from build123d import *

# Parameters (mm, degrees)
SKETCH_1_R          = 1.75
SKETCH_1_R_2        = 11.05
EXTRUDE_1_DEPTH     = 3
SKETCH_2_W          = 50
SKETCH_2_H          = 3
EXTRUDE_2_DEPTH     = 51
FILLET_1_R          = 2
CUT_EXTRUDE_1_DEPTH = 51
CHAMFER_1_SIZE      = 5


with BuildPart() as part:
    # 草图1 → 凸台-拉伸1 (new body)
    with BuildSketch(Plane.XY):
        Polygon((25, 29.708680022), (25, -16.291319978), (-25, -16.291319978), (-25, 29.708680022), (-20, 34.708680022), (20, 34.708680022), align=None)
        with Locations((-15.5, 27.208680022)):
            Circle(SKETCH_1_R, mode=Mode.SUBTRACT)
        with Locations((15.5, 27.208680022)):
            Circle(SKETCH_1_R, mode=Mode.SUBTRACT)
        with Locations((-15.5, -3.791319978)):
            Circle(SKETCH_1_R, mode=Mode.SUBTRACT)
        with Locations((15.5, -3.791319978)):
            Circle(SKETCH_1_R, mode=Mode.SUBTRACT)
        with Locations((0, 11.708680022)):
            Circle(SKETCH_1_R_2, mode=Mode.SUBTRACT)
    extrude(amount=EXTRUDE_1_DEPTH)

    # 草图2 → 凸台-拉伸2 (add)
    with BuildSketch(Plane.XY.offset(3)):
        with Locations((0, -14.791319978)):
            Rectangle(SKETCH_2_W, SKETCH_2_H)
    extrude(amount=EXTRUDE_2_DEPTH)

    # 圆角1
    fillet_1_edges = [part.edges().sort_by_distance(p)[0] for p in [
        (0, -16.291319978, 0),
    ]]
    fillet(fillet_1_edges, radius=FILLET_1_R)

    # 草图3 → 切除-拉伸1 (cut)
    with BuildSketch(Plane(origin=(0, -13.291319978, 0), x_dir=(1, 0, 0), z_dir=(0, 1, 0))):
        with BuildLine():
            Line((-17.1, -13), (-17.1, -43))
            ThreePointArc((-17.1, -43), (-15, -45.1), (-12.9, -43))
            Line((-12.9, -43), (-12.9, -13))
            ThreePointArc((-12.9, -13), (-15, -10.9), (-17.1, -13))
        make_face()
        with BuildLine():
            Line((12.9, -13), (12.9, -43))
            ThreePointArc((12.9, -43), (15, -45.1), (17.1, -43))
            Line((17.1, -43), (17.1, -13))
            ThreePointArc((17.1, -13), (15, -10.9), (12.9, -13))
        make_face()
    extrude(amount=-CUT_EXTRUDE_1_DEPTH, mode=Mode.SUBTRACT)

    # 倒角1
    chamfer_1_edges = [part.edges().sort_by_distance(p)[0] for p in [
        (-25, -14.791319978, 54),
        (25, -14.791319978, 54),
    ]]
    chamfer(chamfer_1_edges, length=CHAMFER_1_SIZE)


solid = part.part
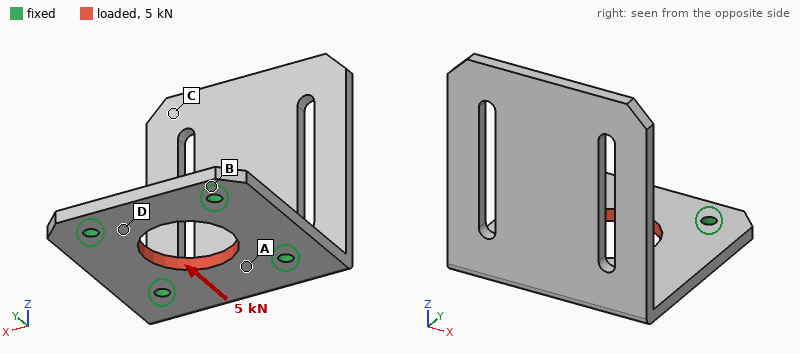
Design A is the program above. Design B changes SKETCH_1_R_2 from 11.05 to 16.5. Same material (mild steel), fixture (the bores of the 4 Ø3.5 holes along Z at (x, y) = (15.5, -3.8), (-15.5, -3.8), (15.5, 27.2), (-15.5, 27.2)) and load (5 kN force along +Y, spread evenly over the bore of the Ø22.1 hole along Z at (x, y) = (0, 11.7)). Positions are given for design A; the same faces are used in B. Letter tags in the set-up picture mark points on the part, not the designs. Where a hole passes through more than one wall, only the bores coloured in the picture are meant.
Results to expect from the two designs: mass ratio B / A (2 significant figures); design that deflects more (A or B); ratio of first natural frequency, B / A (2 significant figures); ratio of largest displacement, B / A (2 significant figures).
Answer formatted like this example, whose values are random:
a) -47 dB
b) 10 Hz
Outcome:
a) 0.89
b) B
c) 0.97
d) 1.4
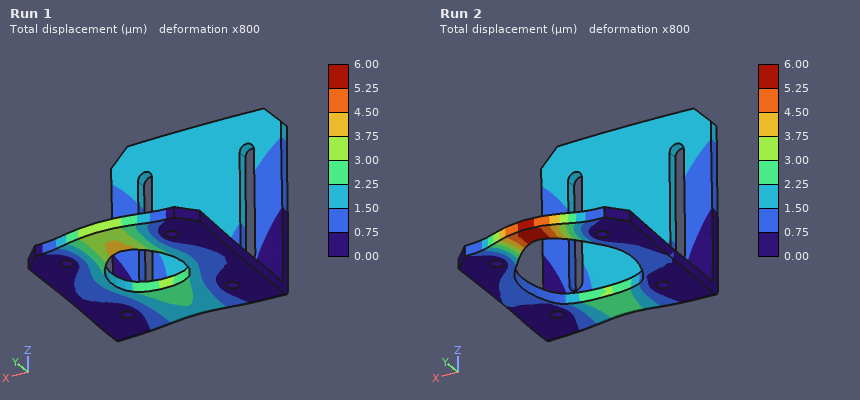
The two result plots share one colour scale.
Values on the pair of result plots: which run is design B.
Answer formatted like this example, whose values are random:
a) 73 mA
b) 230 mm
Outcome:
a) Run 2
